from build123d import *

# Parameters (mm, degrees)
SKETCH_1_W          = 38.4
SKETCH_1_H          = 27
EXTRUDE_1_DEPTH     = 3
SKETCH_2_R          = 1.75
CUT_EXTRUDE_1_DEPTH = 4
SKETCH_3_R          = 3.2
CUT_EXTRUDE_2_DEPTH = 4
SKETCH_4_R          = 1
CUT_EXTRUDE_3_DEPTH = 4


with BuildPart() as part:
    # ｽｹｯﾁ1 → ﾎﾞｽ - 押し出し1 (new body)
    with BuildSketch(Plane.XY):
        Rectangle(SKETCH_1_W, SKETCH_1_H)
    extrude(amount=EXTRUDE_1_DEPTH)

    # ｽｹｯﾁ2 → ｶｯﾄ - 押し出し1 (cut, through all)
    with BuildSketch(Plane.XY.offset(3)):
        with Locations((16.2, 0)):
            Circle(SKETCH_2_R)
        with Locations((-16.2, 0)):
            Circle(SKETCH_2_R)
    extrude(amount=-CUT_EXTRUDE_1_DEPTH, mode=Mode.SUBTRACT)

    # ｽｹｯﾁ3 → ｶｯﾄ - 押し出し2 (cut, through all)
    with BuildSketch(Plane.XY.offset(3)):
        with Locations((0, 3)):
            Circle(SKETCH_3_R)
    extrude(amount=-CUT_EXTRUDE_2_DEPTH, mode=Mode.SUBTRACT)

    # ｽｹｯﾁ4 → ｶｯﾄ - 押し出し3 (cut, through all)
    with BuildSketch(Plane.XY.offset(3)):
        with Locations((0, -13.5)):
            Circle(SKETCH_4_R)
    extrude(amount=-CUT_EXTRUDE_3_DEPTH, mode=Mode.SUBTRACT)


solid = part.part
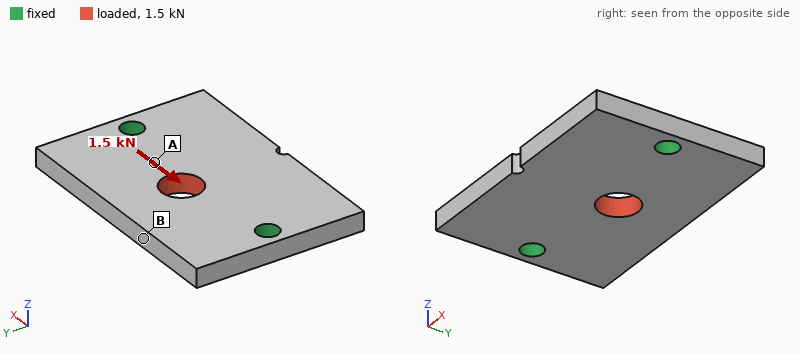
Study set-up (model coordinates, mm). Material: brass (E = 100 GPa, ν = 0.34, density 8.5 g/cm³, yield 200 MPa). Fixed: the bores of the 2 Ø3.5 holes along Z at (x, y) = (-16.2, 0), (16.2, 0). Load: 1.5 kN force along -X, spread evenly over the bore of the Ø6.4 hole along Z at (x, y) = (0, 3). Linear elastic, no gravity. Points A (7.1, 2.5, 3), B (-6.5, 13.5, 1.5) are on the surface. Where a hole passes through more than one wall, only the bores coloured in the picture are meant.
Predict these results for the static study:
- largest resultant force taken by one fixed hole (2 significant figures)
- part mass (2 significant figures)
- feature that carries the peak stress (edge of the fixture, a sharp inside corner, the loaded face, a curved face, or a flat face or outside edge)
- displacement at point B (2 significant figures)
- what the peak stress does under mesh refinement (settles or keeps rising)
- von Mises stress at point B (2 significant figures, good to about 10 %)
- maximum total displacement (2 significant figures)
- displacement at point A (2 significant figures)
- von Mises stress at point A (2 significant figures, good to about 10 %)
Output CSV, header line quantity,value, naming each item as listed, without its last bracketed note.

quantity,value
largest resultant force taken by one fixed hole,760 N
part mass,25 g
feature that carries the peak stress,edge of the fixture
displacement at point B,3.0 µm
what the peak stress does under mesh refinement,keeps rising
von Mises stress at point B,6.6 MPa
maximum total displacement,4.5 µm
displacement at point A,2.5 µm
von Mises stress at point A,28 MPa
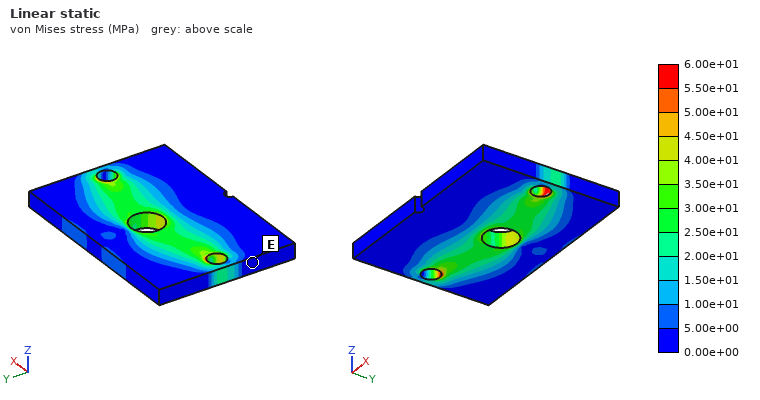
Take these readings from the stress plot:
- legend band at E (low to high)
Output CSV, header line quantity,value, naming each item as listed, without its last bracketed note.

quantity,value
legend band at E,0.00e+00 to 5.00e+00 MPa
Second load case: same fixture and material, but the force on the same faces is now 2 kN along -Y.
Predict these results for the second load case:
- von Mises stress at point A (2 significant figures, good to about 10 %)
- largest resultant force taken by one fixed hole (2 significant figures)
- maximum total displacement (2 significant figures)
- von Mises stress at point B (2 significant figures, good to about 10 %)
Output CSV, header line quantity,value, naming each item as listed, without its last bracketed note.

quantity,value
von Mises stress at point A,29 MPa
largest resultant force taken by one fixed hole,1.0 kN
maximum total displacement,9.8 µm
von Mises stress at point B,29 MPa
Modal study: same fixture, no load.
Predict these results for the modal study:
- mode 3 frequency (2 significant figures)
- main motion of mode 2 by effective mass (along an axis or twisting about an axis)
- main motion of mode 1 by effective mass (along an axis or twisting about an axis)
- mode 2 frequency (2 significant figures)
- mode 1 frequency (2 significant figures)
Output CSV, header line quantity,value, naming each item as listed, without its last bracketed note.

quantity,value
mode 3 frequency,11 kHz
main motion of mode 2 by effective mass,along Z
main motion of mode 1 by effective mass,twisting about X
mode 2 frequency,7000 Hz
mode 1 frequency,5800 Hz
